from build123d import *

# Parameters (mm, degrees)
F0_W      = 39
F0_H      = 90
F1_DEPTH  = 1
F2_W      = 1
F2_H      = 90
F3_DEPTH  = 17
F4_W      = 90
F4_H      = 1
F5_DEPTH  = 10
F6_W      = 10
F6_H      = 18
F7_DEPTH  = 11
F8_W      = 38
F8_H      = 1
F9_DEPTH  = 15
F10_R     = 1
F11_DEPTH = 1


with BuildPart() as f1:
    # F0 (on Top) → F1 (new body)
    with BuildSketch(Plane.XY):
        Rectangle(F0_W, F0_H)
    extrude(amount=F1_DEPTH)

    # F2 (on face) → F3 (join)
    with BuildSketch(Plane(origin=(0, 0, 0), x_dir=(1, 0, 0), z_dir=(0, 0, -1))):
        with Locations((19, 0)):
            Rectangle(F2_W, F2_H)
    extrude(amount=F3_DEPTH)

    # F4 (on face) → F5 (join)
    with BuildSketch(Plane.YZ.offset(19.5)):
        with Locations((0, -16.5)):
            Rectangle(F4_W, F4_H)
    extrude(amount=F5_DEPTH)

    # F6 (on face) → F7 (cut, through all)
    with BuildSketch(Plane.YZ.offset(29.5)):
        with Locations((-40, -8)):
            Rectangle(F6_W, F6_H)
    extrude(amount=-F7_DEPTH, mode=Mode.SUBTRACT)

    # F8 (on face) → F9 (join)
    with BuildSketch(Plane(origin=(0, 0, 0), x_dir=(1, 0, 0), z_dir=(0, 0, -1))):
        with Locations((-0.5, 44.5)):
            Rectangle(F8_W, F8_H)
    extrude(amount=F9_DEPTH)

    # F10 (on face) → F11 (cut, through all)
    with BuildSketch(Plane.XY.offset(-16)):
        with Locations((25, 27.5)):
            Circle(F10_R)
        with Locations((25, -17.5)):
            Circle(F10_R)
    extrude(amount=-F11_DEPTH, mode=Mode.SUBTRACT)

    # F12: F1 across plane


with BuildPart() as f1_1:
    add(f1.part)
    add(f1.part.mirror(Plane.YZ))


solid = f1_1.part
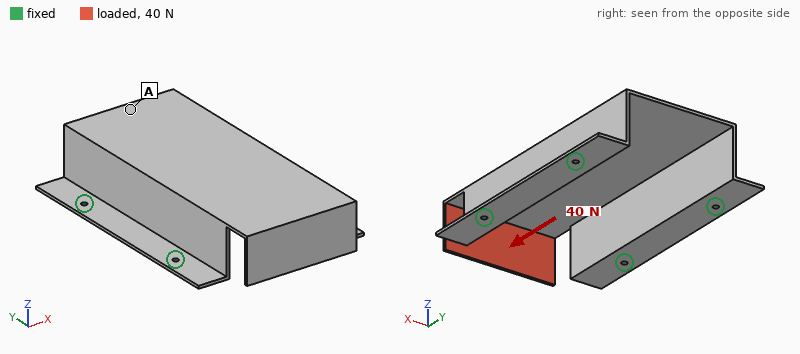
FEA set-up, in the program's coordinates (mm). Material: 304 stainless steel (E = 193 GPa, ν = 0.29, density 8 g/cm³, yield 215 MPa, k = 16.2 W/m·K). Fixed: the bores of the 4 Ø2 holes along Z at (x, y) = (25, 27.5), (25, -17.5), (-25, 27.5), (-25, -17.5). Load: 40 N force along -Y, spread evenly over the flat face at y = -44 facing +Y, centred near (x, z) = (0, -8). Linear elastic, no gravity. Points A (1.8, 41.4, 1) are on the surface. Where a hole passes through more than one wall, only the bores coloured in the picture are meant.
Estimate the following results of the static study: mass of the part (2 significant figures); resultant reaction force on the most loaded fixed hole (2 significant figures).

67 g
13 N
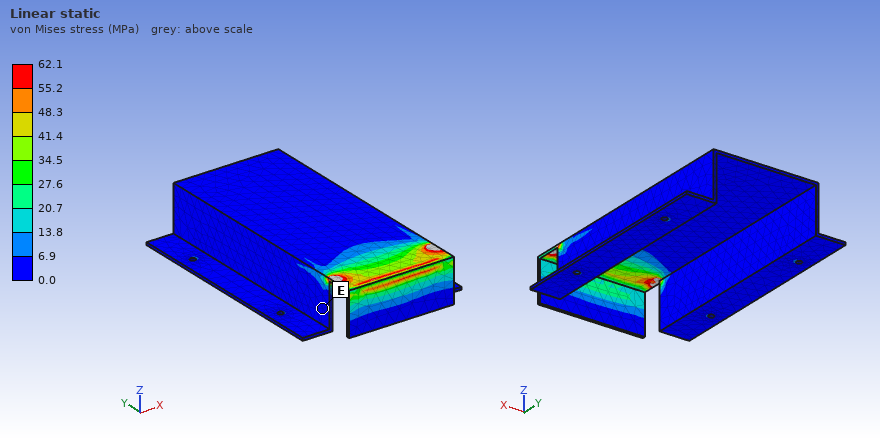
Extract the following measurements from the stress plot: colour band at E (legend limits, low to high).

0.0 to 6.9 MPa
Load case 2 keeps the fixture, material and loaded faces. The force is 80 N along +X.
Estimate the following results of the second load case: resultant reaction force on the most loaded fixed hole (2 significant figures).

83 N
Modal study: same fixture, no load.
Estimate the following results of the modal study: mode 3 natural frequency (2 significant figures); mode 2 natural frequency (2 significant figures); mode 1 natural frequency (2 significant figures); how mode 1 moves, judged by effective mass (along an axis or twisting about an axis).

1900 Hz
1200 Hz
1100 Hz
along X
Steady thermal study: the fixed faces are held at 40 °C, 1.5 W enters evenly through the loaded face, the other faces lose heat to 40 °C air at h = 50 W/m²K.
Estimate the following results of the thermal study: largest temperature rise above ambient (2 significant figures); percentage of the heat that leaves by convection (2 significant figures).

24 K
99 %
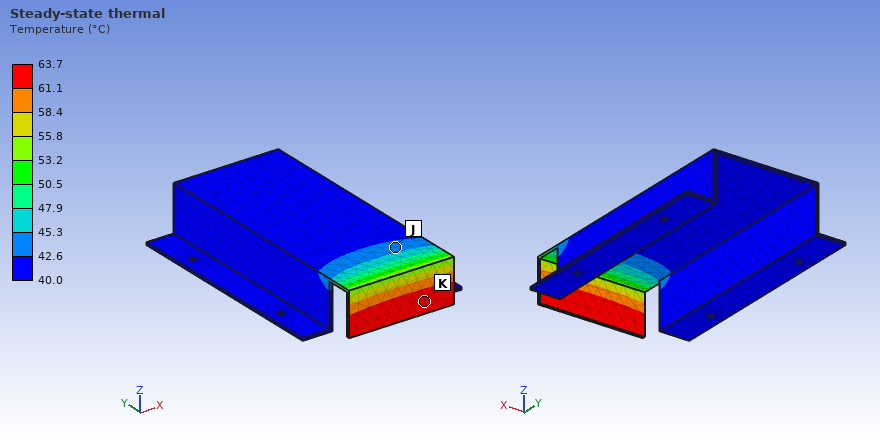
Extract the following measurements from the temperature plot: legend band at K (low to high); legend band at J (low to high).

61.1 to 63.7 °C
42.6 to 45.3 °C
